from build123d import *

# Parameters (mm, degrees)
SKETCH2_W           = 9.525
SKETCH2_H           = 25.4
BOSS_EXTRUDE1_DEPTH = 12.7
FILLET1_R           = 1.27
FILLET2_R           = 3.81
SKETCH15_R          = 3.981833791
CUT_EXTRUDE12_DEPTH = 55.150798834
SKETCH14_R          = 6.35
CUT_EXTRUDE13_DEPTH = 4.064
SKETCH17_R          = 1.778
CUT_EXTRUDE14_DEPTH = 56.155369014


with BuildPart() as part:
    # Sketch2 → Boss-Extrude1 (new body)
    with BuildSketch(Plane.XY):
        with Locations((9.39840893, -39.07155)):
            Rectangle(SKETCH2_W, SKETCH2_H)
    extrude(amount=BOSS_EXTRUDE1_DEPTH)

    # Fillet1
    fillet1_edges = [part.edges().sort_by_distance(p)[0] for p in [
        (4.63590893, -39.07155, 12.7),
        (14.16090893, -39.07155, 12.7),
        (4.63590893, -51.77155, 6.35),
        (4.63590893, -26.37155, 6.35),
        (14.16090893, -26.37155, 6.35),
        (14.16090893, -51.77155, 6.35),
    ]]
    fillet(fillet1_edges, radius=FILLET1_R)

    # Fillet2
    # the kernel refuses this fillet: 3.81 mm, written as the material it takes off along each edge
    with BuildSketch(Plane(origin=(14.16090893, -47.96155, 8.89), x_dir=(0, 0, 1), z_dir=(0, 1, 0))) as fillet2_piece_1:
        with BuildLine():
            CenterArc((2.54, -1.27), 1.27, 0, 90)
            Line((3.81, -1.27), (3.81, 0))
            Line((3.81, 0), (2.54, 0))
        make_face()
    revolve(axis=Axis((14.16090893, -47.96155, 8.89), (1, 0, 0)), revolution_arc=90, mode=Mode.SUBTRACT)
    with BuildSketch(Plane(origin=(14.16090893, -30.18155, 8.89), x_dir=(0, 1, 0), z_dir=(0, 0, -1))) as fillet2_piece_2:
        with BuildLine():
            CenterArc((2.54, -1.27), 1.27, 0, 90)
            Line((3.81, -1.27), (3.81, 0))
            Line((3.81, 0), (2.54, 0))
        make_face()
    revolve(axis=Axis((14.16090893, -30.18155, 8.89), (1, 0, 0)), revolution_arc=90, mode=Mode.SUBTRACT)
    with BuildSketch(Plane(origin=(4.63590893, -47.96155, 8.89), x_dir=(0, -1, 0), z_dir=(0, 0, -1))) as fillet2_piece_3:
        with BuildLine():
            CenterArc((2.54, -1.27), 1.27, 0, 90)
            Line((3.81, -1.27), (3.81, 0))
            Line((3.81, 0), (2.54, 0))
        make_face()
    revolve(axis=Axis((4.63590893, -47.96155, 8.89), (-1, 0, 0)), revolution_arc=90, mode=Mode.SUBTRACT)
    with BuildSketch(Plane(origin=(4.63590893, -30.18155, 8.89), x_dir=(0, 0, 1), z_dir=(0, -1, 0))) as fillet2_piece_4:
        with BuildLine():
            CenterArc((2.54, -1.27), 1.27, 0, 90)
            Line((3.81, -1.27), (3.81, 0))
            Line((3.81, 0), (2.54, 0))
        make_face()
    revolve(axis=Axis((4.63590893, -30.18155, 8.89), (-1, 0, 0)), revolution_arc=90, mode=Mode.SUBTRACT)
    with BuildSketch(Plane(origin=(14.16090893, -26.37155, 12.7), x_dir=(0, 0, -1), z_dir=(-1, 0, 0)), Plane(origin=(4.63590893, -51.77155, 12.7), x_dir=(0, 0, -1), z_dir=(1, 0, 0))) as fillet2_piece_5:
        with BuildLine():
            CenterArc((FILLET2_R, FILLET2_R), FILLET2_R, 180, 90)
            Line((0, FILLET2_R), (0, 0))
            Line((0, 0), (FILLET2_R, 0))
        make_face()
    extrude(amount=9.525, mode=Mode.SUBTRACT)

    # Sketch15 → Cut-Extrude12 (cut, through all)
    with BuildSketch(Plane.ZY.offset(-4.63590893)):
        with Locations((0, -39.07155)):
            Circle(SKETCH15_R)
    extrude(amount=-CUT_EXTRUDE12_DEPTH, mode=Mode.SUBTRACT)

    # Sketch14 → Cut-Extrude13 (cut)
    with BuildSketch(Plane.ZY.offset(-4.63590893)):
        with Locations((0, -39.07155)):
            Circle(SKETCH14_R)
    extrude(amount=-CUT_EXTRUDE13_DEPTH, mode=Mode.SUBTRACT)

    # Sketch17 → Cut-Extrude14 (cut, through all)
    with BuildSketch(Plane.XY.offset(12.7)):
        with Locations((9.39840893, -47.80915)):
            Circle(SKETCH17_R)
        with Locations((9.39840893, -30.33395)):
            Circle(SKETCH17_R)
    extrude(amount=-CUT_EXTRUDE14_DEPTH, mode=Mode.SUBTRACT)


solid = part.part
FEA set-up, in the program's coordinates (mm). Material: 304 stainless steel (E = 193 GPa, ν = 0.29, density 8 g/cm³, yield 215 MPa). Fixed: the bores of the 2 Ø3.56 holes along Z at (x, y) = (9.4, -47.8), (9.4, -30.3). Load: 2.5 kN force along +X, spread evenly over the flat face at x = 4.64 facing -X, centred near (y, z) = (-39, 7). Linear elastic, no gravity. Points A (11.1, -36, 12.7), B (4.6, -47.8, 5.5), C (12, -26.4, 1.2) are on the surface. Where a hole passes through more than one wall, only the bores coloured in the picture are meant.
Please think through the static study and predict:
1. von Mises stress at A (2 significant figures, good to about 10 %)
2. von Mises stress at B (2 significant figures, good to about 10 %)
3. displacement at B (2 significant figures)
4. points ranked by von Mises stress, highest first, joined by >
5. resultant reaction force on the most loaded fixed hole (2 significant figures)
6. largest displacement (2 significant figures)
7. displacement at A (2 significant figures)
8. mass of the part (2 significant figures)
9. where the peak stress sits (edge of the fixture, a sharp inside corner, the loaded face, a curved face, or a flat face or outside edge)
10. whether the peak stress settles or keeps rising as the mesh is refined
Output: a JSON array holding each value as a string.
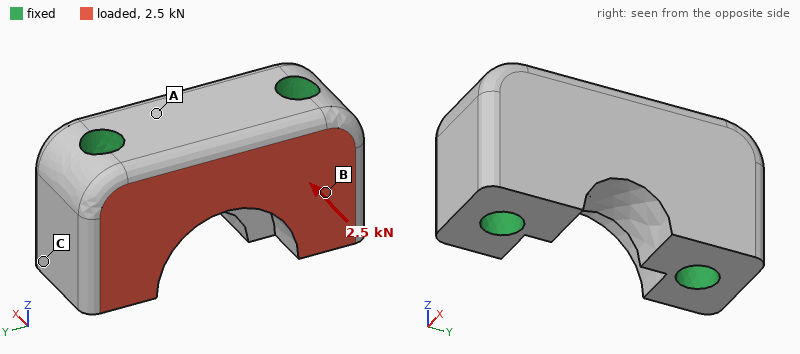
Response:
["8.3 MPa", "15 MPa", "0.26 µm", "B > A > C", "1.3 kN", "0.81 µm", "0.54 µm", "19 g", "edge of the fixture", "keeps rising"]
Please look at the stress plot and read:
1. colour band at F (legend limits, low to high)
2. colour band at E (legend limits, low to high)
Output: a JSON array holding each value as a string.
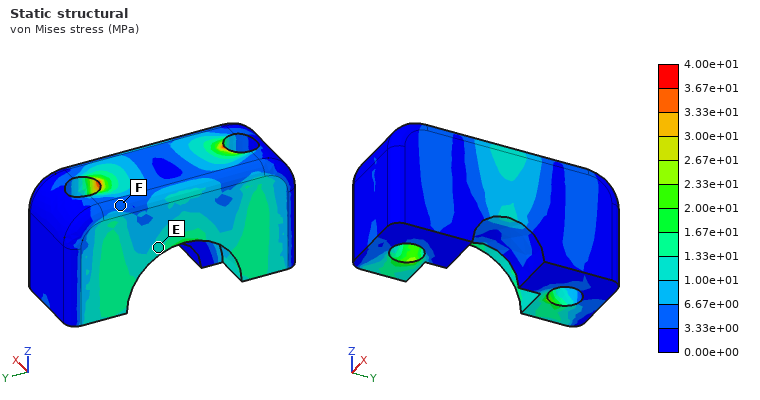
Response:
["3.33e+00 to 6.67e+00 MPa", "1.00e+01 to 1.33e+01 MPa"]
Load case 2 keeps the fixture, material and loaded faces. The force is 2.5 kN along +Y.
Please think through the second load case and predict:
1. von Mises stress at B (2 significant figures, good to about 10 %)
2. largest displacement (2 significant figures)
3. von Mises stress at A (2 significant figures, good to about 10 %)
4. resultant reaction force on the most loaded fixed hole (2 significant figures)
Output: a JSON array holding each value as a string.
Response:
["23 MPa", "1.2 µm", "4.3 MPa", "1.3 kN"]
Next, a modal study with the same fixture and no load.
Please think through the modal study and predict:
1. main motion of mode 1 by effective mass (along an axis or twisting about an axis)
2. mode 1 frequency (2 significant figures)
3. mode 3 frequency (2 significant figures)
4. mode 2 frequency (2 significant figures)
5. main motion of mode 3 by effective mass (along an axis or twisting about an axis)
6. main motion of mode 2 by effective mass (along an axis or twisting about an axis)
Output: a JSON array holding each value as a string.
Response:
["along X", "76 kHz", "100 kHz", "90 kHz", "twisting about Y", "along Z"]
